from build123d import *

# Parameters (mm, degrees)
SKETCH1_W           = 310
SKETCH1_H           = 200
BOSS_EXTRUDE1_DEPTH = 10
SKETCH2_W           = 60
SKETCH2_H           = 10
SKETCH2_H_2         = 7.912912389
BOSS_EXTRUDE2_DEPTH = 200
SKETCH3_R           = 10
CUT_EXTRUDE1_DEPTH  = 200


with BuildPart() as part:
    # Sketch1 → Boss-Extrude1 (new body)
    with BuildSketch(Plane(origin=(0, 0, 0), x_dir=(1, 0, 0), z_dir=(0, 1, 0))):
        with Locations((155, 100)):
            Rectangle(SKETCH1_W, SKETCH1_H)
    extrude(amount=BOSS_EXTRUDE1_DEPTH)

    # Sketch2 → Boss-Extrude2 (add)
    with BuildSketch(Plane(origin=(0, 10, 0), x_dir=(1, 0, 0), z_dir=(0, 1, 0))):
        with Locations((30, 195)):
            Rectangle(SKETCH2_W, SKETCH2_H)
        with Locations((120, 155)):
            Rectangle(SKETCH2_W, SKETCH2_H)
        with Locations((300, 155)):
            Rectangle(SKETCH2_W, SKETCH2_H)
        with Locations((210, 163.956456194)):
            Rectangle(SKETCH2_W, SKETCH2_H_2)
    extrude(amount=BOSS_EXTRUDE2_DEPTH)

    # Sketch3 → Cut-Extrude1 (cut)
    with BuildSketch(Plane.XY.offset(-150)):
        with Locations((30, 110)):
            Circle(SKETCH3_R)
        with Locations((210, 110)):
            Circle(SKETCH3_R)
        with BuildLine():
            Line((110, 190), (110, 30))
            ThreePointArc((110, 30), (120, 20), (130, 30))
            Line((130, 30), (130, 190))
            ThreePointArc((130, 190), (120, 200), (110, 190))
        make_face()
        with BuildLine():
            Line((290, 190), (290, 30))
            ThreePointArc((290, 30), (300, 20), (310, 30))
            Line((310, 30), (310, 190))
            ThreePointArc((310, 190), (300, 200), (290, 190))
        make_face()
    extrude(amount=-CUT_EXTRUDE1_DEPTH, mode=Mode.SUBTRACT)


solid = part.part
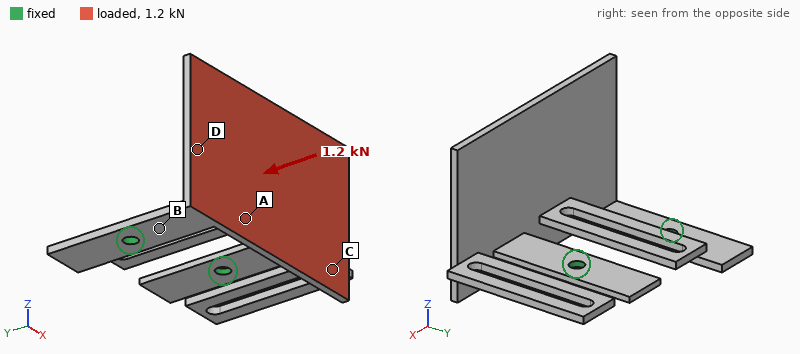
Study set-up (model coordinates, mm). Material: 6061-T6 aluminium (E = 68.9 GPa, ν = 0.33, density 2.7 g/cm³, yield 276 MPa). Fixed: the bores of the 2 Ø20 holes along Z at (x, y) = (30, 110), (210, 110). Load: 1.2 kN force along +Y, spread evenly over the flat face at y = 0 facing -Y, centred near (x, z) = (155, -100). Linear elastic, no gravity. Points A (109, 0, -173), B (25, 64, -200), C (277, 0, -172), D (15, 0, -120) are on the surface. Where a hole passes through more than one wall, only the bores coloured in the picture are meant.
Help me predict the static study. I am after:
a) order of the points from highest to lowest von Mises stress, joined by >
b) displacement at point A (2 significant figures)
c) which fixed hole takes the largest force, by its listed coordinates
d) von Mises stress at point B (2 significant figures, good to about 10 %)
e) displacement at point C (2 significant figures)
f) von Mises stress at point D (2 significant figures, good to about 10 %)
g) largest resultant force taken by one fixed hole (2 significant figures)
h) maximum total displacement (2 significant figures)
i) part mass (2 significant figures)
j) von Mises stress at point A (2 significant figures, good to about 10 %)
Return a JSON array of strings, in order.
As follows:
["B > A > D > C", "0.76 mm", "(210, 110)", "40 MPa", "0.94 mm", "11 MPa", "1.4 kN", "3.1 mm", "2.7 kg", "17 MPa"]
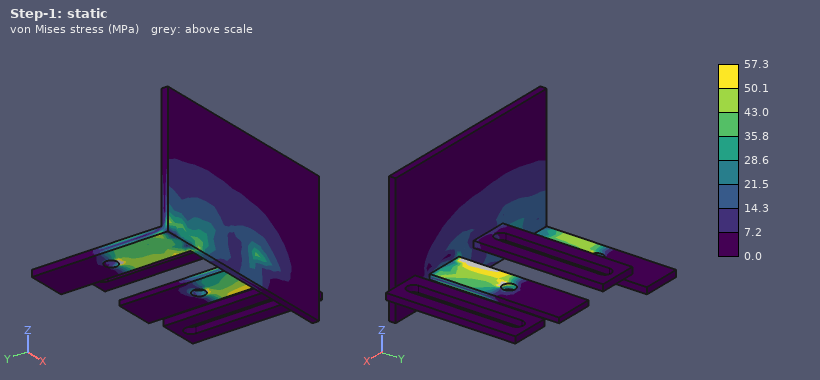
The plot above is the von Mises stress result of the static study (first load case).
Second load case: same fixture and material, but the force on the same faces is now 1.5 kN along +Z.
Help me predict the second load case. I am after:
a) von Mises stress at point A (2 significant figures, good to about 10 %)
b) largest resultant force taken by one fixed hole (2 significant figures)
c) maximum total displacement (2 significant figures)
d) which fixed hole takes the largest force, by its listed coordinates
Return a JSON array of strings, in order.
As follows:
["15 MPa", "1.1 kN", "2.7 mm", "(210, 110)"]
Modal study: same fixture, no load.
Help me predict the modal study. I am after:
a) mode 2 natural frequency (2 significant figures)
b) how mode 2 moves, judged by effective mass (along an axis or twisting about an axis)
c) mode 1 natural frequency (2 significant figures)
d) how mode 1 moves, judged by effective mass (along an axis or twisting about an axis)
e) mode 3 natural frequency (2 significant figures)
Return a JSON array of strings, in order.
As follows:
["140 Hz", "along Z", "78 Hz", "along Y", "170 Hz"]
